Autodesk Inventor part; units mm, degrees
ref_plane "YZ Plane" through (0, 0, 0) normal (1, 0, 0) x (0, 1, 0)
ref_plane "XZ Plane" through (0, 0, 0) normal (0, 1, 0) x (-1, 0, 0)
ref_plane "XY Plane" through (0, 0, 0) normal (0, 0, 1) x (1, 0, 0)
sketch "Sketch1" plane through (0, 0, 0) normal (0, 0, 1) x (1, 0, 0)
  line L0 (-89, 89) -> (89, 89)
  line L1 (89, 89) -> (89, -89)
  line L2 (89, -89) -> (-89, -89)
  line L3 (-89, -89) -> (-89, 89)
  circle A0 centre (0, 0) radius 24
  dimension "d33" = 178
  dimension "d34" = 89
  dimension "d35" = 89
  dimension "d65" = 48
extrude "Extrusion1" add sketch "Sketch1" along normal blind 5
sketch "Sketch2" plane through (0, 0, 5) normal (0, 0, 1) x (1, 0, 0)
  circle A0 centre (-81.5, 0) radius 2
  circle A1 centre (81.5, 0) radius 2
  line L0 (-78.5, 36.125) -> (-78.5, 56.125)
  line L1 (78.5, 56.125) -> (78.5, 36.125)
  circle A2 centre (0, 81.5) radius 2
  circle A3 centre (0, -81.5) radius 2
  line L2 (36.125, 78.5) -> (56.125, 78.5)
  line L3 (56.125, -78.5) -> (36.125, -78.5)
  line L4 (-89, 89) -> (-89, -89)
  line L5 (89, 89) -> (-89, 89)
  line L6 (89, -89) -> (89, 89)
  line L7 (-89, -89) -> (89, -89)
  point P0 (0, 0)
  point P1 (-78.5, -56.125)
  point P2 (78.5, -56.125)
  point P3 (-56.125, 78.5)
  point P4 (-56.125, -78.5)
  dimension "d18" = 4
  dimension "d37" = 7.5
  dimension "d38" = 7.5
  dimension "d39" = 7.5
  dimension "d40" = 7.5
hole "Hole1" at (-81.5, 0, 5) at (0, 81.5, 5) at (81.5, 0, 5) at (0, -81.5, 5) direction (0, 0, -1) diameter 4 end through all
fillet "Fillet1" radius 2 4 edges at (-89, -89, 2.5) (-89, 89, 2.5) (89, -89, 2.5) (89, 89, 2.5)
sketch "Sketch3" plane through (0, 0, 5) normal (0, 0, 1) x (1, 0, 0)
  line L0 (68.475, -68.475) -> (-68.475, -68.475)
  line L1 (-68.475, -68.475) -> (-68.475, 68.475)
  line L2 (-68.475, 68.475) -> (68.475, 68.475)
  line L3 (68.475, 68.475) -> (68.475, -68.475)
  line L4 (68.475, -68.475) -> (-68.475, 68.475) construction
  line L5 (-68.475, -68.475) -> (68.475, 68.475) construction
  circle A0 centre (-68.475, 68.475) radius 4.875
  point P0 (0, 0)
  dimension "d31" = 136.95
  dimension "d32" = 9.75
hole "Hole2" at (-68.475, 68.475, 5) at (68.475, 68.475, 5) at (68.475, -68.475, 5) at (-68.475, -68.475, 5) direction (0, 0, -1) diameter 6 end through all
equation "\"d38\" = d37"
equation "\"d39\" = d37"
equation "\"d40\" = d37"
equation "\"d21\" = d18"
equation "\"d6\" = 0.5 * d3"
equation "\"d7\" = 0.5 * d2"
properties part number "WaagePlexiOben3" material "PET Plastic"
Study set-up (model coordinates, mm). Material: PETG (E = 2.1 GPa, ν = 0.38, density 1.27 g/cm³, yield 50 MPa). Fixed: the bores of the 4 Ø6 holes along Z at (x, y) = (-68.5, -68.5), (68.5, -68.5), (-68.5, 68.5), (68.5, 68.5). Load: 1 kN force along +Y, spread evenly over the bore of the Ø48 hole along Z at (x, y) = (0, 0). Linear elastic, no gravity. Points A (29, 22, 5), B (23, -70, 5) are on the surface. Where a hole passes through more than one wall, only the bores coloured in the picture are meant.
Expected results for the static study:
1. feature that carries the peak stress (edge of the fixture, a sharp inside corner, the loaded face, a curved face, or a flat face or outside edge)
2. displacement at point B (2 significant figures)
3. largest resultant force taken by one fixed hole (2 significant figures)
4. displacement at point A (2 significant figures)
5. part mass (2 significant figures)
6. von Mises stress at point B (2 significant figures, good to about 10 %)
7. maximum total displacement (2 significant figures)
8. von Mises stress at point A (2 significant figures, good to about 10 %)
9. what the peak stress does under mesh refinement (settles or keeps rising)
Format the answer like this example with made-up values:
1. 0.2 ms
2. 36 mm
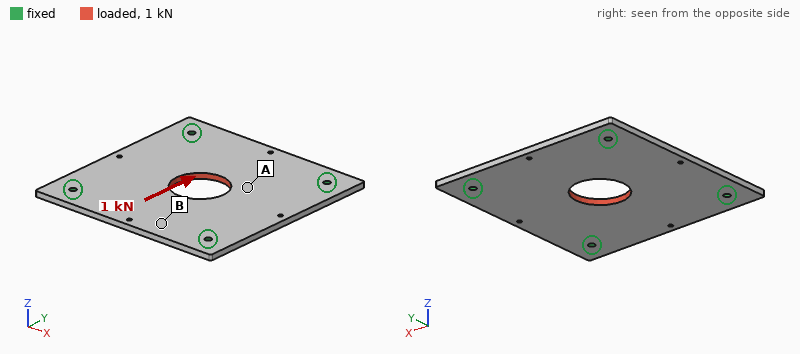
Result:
1. edge of the fixture
2. 51 µm
3. 270 N
4. 53 µm
5. 190 g
6. 0.56 MPa
7. 73 µm
8. 1.2 MPa
9. keeps rising
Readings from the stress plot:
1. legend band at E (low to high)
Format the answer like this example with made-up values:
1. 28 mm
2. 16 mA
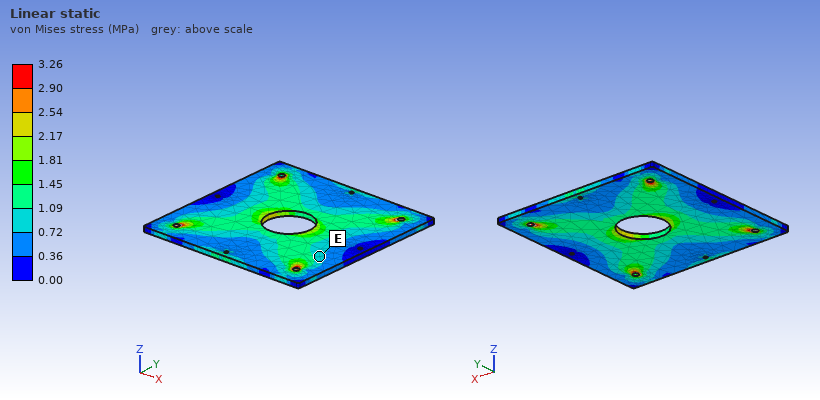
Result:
1. 0.72 to 1.09 MPa
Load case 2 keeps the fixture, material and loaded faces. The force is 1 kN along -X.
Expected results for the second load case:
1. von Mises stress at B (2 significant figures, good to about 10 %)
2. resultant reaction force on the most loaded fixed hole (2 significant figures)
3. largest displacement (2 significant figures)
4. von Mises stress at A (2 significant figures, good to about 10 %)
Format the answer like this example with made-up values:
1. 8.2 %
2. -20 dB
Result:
1. 0.57 MPa
2. 270 N
3. 73 µm
4. 1.2 MPa
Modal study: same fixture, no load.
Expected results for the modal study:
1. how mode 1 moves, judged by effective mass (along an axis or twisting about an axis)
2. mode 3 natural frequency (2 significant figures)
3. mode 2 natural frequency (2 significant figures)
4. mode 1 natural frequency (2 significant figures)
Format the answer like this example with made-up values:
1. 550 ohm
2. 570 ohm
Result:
1. along Z
2. 370 Hz
3. 370 Hz
4. 240 Hz
